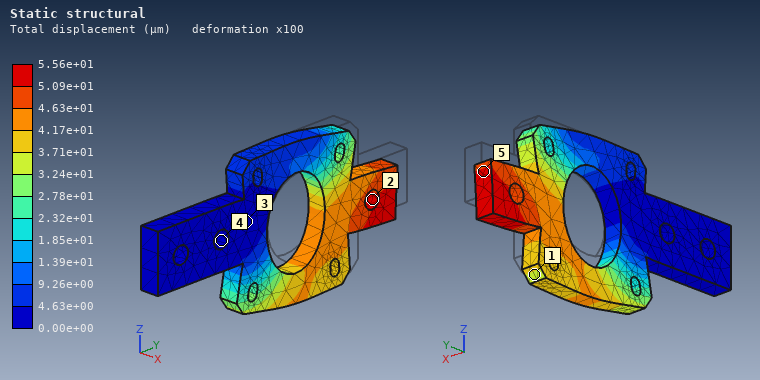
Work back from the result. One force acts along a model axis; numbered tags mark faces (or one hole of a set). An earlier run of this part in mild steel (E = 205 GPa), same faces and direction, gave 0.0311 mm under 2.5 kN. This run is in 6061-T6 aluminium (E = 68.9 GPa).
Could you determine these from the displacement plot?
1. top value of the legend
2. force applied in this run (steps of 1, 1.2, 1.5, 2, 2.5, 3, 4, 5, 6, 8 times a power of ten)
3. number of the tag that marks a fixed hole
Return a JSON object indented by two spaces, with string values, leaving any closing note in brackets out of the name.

{
  "top value of the legend": "5.56e+01 µm",
  "force applied in this run": "1.5 kN",
  "number of the tag that marks a fixed hole": "4"
}
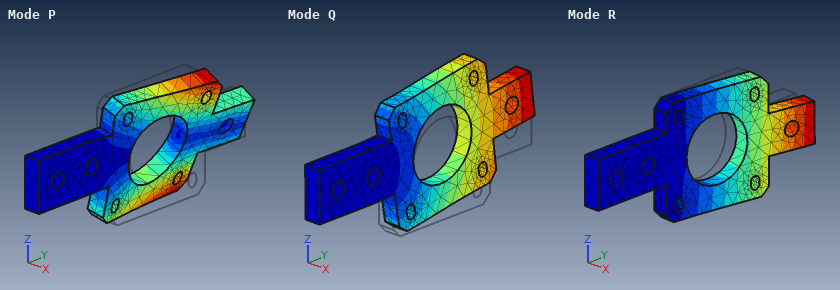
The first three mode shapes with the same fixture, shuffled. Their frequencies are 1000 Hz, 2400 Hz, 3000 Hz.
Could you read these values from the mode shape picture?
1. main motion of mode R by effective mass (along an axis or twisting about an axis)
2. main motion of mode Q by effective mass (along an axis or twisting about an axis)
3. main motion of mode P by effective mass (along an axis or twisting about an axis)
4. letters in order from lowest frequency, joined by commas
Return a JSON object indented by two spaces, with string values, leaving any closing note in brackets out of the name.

{
  "main motion of mode R by effective mass": "along X",
  "main motion of mode Q by effective mass": "along Z",
  "main motion of mode P by effective mass": "twisting about Y",
  "letters in order from lowest frequency, joined by commas": "R, Q, P"
}
